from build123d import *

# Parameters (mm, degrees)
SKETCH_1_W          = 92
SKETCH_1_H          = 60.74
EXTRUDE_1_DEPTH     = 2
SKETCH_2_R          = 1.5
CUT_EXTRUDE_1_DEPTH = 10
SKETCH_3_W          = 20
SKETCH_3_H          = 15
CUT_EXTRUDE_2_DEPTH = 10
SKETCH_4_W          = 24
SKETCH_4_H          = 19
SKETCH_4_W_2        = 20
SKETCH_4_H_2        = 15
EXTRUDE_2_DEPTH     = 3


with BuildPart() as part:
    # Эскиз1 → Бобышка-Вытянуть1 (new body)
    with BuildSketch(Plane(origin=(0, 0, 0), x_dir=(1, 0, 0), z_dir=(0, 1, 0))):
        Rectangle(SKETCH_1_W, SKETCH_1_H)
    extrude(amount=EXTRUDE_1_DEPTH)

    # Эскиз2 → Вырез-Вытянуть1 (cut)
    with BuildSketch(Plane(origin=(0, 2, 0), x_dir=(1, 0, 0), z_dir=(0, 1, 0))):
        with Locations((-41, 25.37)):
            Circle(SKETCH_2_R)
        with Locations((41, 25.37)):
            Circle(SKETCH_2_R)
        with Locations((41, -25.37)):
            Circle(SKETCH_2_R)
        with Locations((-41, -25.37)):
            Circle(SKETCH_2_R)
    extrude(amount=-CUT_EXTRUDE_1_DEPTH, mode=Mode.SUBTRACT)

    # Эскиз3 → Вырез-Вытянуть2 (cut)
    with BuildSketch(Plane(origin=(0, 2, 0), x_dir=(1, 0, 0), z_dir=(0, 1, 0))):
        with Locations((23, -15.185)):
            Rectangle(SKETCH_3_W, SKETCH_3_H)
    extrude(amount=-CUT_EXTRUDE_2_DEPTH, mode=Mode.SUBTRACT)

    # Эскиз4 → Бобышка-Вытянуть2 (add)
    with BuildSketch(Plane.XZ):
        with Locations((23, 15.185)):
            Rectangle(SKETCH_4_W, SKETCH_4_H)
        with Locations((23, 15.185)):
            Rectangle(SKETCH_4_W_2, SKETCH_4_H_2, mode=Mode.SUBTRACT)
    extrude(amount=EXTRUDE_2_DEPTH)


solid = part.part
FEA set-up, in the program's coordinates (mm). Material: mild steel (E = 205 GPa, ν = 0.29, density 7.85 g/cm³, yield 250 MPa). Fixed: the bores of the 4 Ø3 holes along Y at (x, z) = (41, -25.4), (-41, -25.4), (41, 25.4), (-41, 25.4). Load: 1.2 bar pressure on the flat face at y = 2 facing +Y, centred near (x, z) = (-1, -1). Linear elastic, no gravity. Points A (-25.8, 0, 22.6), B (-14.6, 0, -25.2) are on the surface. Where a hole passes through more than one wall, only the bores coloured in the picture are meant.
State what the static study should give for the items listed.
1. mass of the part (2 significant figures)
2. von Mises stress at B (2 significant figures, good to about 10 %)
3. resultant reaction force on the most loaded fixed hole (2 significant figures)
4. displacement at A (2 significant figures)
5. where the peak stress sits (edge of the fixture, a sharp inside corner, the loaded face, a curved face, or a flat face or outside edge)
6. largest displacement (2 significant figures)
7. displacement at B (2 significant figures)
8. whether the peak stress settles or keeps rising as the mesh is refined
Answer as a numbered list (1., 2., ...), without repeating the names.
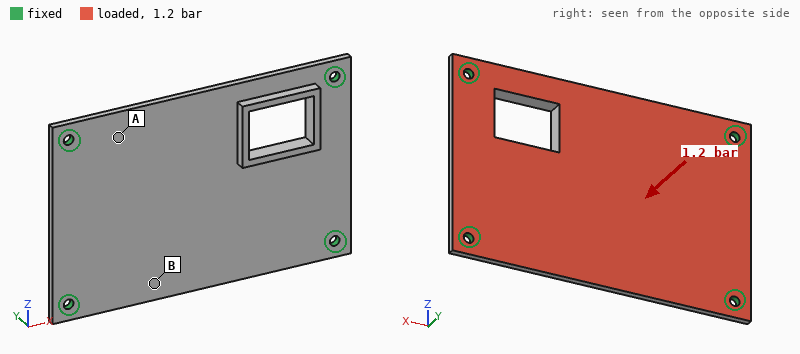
1. 86 g
2. 45 MPa
3. 170 N
4. 0.057 mm
5. edge of the fixture
6. 0.14 mm
7. 0.11 mm
8. keeps rising
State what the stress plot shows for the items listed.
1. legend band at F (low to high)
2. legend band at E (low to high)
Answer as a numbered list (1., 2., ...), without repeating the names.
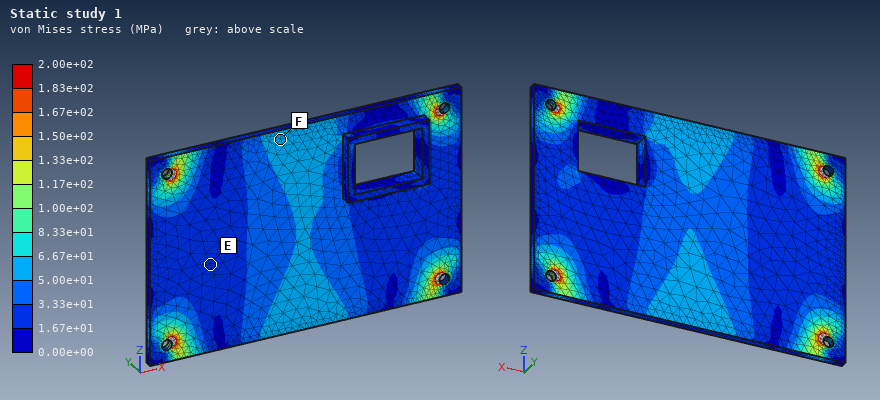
1. 5.00e+01 to 6.67e+01 MPa
2. 1.67e+01 to 3.33e+01 MPa
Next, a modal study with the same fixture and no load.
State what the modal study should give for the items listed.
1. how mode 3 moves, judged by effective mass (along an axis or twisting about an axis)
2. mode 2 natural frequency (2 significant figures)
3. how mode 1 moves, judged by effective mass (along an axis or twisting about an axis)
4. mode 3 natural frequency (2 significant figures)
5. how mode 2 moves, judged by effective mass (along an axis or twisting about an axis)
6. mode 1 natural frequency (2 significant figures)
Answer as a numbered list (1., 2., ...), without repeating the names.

1. twisting about Z
2. 2100 Hz
3. along Y
4. 3400 Hz
5. twisting about X
6. 1300 Hz
